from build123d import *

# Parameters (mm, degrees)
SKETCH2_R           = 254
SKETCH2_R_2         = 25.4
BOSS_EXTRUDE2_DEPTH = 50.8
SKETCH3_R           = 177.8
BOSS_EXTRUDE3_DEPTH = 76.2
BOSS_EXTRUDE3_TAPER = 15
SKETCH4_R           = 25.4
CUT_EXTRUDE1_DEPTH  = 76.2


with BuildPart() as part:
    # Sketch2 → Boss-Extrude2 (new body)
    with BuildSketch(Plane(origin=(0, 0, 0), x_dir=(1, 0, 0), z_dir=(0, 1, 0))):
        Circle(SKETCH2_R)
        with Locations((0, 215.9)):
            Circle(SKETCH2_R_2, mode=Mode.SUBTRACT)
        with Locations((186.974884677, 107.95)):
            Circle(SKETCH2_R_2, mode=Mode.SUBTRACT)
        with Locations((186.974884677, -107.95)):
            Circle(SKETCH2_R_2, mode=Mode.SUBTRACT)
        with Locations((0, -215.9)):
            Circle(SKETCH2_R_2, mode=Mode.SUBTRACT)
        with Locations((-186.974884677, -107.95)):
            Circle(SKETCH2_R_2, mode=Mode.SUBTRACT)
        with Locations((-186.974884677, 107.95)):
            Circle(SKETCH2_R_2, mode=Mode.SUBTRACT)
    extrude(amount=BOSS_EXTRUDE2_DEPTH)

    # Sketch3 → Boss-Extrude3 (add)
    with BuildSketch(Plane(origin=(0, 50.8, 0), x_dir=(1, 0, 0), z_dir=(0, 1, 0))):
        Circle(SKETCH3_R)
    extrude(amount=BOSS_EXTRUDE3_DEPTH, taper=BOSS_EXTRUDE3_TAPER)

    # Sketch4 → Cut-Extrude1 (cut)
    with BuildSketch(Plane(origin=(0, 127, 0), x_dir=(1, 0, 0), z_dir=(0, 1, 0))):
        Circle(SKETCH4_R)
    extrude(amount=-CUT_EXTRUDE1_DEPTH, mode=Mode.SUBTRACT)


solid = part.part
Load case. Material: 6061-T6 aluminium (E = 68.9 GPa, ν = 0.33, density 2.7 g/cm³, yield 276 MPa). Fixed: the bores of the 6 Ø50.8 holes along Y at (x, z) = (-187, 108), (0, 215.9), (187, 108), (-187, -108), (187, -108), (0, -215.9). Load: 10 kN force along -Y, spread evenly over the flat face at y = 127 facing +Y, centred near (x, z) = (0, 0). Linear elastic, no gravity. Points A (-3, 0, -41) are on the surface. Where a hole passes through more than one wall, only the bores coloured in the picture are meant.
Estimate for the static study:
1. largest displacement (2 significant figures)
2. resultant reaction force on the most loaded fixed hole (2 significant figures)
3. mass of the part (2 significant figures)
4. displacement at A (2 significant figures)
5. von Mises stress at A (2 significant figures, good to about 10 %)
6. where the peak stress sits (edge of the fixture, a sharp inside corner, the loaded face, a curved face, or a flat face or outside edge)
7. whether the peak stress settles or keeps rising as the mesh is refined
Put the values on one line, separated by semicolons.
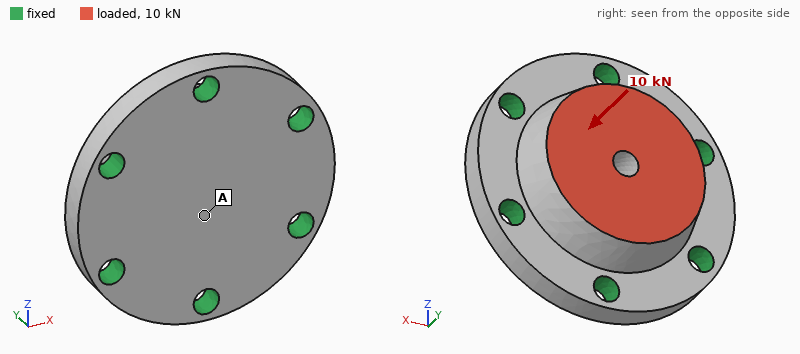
1.4 µm; 1.9 kN; 44 kg; 1.2 µm; 0.22 MPa; edge of the fixture; keeps rising
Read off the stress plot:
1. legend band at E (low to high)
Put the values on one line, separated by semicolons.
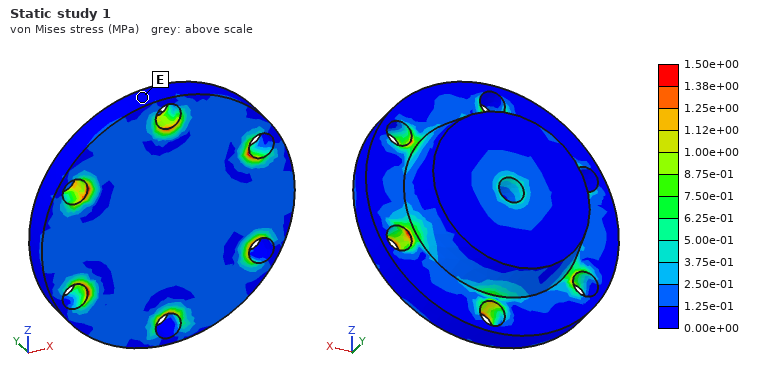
0.00e+00 to 1.25e-01 MPa
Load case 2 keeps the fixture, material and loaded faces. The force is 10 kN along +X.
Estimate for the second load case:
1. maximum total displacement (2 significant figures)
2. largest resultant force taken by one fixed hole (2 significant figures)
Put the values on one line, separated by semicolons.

1.3 µm; 2.6 kN
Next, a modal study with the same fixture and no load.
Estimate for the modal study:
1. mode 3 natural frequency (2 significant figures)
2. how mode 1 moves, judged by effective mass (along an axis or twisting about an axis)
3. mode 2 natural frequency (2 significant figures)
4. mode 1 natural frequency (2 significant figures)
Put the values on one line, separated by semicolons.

3900 Hz; along Y; 3900 Hz; 2800 Hz
